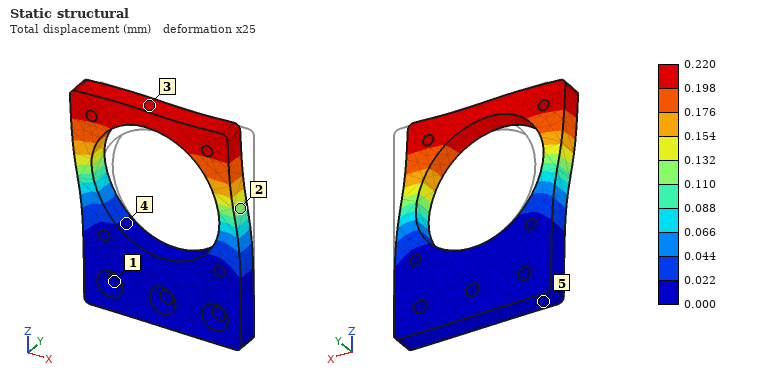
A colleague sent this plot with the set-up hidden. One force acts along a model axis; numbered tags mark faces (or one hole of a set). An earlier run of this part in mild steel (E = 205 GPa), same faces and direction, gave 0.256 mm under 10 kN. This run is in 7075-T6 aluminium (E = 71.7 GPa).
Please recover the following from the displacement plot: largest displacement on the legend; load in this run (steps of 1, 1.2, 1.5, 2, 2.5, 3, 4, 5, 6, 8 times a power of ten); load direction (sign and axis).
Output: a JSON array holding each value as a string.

["0.220 mm", "3 kN", "-X"]
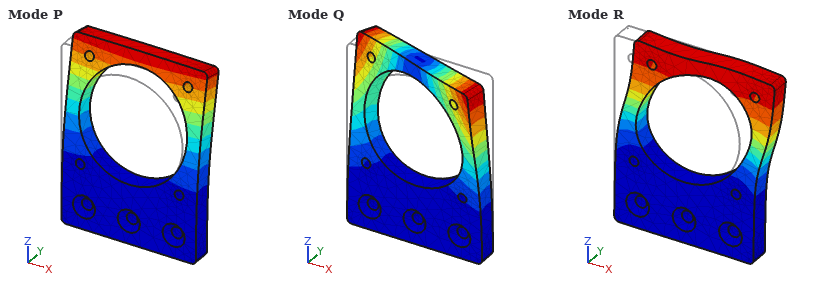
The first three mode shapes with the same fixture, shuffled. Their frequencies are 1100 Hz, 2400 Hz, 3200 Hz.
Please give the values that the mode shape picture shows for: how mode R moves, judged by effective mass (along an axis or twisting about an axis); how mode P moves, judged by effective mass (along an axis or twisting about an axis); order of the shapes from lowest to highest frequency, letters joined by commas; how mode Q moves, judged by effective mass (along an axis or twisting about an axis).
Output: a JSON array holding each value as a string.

["along X", "along Y", "P, Q, R", "twisting about Z"]
